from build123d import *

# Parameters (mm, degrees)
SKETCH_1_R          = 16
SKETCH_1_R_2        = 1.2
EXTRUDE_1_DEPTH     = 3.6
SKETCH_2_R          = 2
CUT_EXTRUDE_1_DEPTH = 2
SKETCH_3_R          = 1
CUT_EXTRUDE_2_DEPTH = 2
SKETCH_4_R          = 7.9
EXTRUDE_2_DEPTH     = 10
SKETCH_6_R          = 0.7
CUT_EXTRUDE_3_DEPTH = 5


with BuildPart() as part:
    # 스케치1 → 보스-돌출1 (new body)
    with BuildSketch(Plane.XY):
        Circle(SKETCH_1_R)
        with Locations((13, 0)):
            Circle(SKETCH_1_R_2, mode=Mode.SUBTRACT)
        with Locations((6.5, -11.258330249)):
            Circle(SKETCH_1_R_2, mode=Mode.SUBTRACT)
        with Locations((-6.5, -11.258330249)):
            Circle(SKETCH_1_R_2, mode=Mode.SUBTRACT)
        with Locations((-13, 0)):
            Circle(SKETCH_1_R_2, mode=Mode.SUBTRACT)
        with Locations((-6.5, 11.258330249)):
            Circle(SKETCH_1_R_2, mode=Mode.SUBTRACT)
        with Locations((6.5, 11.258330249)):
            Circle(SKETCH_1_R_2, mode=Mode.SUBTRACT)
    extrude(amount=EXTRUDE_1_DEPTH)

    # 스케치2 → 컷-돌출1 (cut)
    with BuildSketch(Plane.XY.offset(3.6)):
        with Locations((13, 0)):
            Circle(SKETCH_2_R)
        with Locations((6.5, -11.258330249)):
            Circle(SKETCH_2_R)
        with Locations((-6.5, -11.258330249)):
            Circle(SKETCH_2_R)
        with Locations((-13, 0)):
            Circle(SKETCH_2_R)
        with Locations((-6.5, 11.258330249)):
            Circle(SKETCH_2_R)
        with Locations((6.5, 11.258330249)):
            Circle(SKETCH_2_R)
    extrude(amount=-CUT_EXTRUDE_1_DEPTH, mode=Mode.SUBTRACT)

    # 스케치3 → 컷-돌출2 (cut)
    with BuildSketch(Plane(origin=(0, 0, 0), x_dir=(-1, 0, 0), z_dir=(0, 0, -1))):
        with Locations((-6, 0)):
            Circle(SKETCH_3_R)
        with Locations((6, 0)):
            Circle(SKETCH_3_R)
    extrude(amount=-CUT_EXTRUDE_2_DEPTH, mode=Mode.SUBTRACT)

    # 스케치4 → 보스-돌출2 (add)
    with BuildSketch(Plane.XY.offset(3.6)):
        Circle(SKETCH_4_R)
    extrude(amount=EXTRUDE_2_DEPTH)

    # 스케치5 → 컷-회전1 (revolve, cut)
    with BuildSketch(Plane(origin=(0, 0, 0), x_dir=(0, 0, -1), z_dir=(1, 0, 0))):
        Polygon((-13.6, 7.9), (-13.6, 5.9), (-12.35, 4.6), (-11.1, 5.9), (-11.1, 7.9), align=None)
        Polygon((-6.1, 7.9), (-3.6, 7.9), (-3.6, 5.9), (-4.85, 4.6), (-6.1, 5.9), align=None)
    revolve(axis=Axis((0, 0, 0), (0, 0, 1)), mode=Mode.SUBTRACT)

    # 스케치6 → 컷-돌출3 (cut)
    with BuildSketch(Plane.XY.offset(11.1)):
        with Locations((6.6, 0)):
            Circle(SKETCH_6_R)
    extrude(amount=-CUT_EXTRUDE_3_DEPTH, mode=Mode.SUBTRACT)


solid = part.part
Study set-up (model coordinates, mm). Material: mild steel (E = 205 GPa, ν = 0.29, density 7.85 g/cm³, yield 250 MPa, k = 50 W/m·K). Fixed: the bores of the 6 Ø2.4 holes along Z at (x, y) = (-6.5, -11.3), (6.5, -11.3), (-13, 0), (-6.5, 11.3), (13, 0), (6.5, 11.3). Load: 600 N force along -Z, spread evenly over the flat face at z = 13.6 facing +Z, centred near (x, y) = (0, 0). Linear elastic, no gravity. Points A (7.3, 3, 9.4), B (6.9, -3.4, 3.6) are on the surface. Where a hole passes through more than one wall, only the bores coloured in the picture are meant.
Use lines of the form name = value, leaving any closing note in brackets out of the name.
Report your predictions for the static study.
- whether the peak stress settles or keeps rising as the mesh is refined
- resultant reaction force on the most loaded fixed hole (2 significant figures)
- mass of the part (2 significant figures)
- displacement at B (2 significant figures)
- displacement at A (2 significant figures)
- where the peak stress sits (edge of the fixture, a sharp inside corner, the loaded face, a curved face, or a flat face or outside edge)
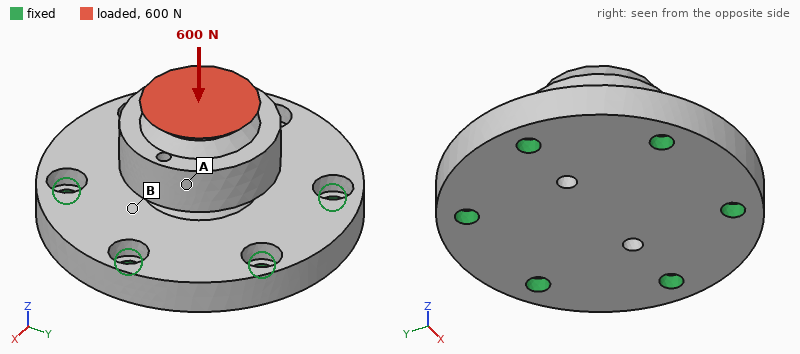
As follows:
whether the peak stress settles or keeps rising as the mesh is refined = keeps rising
resultant reaction force on the most loaded fixed hole = 160 N
mass of the part = 32 g
displacement at B = 1.2 µm
displacement at A = 2.0 µm
where the peak stress sits = edge of the fixture
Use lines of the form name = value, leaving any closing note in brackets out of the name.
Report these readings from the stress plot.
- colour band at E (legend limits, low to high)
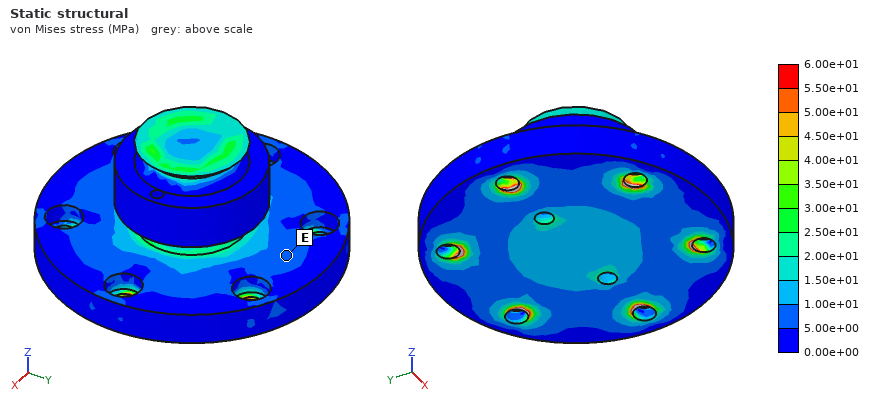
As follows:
colour band at E = 5.00e+00 to 1.00e+01 MPa
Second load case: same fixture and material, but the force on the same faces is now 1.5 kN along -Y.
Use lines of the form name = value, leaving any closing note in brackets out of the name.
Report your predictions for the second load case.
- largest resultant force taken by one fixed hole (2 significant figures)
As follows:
largest resultant force taken by one fixed hole = 650 N
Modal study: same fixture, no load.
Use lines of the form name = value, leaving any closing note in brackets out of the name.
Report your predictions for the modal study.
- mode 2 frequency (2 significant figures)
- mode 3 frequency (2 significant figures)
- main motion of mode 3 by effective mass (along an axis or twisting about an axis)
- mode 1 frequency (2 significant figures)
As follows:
mode 2 frequency = 21 kHz
mode 3 frequency = 22 kHz
main motion of mode 3 by effective mass = along Z
mode 1 frequency = 20 kHz
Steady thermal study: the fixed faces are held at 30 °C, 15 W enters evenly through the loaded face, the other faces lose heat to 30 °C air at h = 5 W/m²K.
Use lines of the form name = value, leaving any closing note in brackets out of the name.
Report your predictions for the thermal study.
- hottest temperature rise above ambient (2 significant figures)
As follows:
hottest temperature rise above ambient = 58 K
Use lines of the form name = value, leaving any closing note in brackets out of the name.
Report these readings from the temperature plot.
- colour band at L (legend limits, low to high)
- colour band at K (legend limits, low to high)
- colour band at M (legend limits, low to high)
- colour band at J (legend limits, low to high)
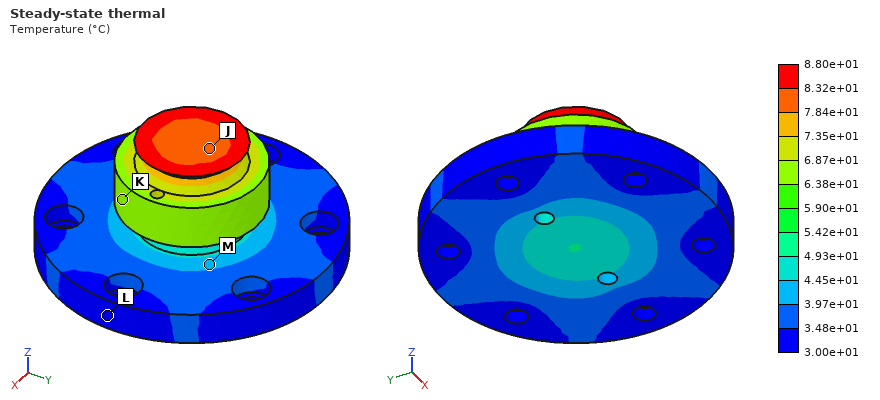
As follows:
colour band at L = 3.00e+01 to 3.48e+01 °C
colour band at K = 6.38e+01 to 6.87e+01 °C
colour band at M = 3.97e+01 to 4.45e+01 °C
colour band at J = 7.84e+01 to 8.32e+01 °C
